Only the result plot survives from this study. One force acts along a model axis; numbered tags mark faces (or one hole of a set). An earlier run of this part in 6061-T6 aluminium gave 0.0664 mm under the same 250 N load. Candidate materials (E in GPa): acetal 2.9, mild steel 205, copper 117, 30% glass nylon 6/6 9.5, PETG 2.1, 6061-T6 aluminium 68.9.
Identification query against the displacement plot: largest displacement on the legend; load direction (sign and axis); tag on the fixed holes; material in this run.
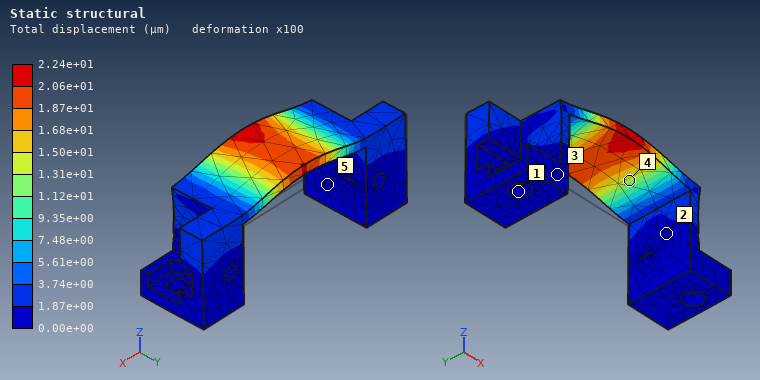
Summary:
2.24e+01 µm
+Z
1
mild steel
